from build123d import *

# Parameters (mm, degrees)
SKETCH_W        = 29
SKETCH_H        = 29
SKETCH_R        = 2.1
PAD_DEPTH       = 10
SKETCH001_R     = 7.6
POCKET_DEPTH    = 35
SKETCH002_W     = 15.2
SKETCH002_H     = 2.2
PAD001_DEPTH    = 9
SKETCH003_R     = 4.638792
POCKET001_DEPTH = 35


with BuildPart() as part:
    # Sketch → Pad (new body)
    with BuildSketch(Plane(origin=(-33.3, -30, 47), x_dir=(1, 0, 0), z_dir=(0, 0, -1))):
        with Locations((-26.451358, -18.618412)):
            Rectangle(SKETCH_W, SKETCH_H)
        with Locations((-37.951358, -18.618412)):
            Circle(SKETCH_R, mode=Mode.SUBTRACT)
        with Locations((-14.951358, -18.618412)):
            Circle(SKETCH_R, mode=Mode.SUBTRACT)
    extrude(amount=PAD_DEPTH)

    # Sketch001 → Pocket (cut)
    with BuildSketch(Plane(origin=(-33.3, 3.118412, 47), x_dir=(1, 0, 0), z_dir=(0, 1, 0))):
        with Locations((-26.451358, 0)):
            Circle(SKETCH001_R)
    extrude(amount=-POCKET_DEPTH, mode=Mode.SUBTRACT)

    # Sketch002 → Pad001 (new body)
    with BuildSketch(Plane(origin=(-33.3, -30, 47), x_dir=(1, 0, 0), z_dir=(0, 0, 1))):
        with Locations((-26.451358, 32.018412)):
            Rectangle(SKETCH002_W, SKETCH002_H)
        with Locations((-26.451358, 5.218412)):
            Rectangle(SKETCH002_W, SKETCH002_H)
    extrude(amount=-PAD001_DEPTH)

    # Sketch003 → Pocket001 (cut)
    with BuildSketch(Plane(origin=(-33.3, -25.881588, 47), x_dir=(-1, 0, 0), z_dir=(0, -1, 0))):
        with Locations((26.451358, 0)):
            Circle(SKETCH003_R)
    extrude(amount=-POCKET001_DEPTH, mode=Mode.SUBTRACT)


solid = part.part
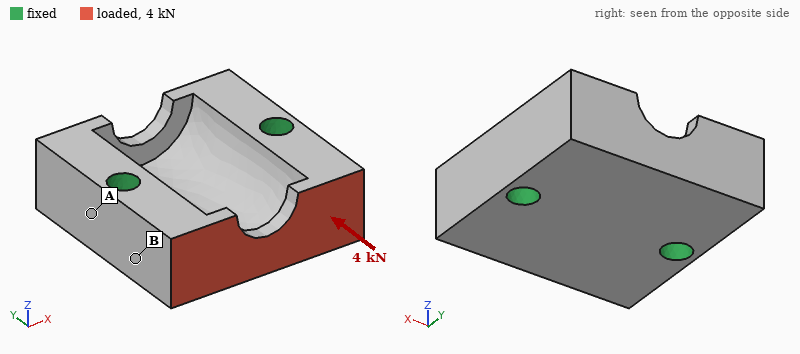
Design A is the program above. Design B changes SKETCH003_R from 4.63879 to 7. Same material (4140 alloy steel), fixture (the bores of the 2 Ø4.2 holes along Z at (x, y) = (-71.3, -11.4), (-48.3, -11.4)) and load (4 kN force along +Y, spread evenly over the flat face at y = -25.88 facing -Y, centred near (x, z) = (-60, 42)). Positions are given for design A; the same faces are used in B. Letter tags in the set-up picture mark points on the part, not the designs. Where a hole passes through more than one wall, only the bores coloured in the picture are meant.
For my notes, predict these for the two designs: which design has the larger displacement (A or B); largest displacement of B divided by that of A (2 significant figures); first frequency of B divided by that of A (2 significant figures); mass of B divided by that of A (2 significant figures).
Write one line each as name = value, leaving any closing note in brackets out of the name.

which design has the larger displacement = A
largest displacement of B divided by that of A = 0.40
first frequency of B divided by that of A = 1.0
mass of B divided by that of A = 0.97
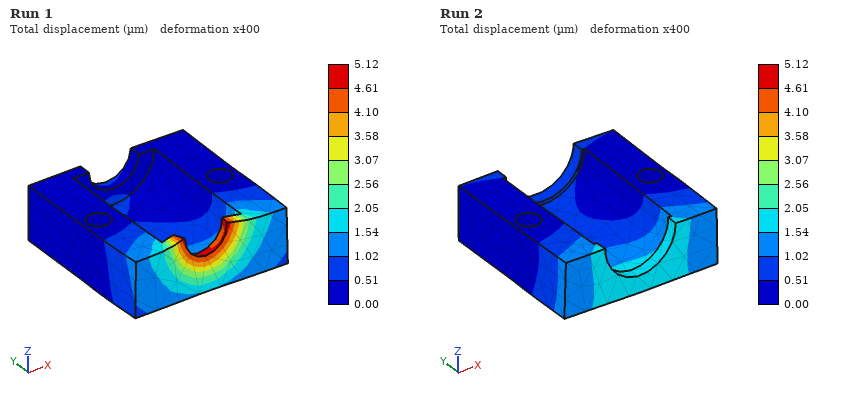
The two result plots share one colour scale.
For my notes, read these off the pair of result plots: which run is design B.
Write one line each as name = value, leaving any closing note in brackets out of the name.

which run is design B = Run 2
